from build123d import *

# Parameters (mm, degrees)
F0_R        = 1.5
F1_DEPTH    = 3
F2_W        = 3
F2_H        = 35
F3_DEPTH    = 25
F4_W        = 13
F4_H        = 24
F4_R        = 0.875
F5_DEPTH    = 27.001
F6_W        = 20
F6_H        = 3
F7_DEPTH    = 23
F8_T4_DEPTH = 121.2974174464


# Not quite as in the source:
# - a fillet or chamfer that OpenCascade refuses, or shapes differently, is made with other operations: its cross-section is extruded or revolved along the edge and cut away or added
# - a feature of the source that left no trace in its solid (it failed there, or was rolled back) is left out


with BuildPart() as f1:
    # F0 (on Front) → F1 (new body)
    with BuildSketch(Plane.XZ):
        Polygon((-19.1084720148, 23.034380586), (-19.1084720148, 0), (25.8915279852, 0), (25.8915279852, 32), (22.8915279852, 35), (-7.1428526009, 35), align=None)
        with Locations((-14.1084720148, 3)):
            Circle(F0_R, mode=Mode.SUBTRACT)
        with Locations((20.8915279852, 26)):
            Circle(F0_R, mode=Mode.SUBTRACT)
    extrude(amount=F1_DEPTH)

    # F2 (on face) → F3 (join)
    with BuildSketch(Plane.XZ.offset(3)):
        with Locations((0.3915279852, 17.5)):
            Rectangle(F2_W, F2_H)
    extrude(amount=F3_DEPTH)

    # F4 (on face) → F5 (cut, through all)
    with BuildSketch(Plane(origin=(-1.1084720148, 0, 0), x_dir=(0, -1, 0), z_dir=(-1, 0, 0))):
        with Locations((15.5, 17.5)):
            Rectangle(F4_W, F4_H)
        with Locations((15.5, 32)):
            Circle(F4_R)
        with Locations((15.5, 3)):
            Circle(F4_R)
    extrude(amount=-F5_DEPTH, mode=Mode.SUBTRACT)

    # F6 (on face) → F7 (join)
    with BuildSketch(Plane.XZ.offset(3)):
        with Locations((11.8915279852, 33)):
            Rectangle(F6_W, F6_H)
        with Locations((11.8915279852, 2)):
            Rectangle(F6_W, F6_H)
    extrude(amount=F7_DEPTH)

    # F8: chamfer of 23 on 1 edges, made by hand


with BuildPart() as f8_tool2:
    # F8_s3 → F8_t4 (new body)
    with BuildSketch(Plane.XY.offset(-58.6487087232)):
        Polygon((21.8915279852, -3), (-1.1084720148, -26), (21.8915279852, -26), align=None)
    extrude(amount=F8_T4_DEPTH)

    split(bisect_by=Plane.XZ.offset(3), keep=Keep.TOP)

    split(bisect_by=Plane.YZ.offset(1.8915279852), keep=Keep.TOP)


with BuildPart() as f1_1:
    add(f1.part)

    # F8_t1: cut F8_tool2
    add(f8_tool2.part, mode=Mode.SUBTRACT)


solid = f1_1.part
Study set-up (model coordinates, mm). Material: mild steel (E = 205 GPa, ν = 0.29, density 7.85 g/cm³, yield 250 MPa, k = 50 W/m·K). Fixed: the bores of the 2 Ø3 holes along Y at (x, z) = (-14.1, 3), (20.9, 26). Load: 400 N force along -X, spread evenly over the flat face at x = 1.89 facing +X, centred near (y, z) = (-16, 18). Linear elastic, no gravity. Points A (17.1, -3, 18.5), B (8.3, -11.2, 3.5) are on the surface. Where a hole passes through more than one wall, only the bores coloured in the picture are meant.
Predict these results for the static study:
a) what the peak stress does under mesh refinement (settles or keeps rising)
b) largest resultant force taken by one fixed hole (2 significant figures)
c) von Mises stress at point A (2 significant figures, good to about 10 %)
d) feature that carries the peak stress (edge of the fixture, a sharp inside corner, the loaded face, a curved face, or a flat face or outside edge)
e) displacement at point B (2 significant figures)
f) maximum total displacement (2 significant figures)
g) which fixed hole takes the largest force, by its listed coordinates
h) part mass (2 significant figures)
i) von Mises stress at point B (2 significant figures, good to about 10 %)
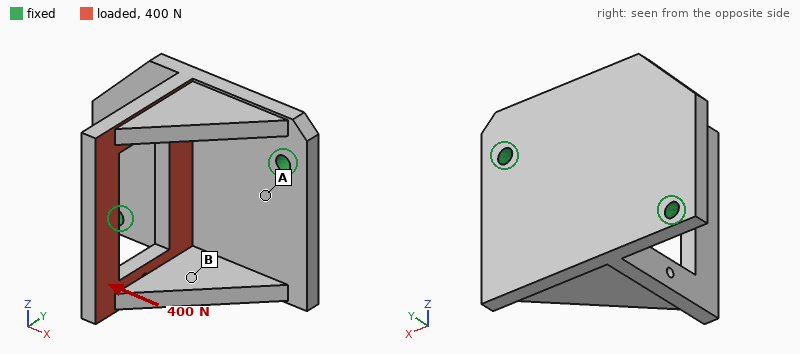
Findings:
keeps rising
270 N
38 MPa
edge of the fixture
27 µm
64 µm
(20.9, 26)
58 g
15 MPa
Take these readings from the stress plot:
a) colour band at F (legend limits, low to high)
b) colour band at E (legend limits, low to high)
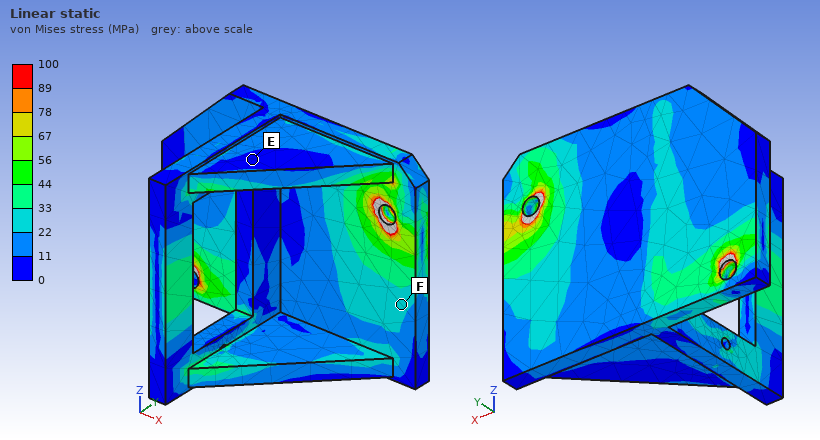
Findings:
22 to 33 MPa
0 to 11 MPa
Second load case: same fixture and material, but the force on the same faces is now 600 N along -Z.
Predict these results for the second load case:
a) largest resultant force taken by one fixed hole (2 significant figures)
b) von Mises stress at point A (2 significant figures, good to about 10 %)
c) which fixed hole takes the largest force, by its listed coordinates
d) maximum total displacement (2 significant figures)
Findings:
380 N
51 MPa
(-14.1, 3)
0.12 mm
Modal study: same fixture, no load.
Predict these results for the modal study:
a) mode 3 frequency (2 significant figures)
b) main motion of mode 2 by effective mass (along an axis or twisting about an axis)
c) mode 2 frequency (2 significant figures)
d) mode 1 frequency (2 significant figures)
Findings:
6100 Hz
along Y
4400 Hz
2400 Hz
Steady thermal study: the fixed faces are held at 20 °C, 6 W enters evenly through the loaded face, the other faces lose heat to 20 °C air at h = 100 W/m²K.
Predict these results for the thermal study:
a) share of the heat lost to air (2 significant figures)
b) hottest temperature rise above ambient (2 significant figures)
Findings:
62 %
25 K
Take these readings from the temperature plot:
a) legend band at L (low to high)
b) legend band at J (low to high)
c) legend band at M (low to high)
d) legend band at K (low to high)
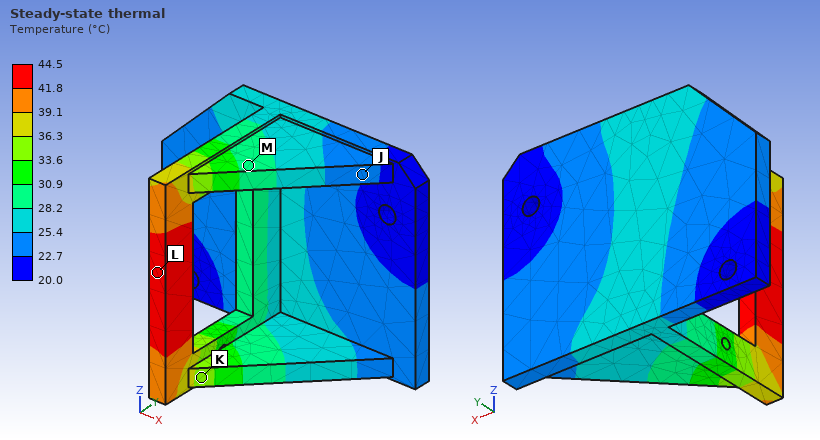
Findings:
41.8 to 44.5 °C
22.7 to 25.4 °C
28.2 to 30.9 °C
33.6 to 36.3 °C
